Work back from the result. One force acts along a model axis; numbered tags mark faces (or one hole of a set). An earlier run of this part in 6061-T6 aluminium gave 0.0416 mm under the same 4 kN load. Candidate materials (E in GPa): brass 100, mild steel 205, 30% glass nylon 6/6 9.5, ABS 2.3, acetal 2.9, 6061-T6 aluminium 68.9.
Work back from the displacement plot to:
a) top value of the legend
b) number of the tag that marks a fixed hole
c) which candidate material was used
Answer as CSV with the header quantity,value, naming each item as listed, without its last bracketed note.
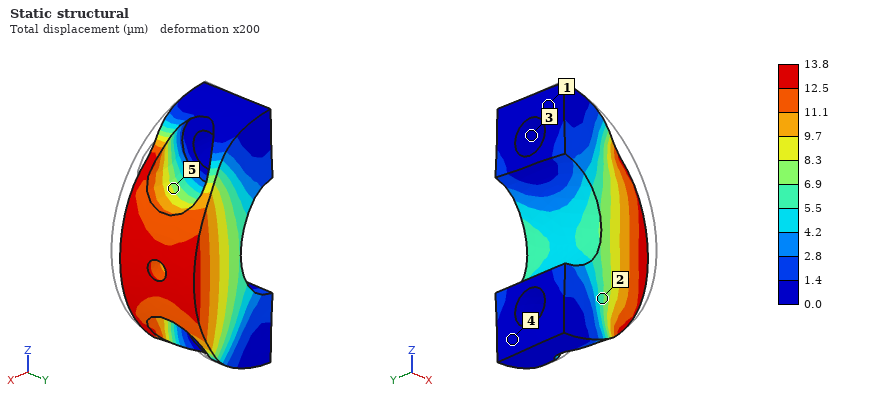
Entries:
quantity,value
top value of the legend,13.8 µm
number of the tag that marks a fixed hole,3
which candidate material was used,mild steel
